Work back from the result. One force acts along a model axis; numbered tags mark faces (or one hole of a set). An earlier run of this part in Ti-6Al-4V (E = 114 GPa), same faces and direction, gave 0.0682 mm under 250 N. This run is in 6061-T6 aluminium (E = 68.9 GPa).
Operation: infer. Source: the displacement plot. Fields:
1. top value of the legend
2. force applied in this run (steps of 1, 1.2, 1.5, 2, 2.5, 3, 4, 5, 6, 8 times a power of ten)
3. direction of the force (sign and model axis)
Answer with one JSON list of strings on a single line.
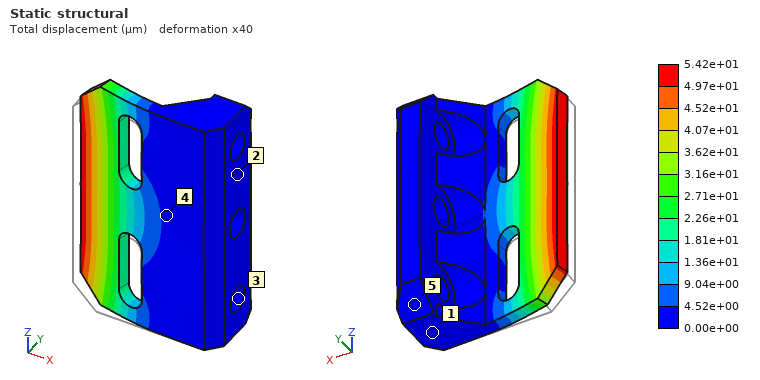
["5.42e+01 µm", "120 N", "+Y"]
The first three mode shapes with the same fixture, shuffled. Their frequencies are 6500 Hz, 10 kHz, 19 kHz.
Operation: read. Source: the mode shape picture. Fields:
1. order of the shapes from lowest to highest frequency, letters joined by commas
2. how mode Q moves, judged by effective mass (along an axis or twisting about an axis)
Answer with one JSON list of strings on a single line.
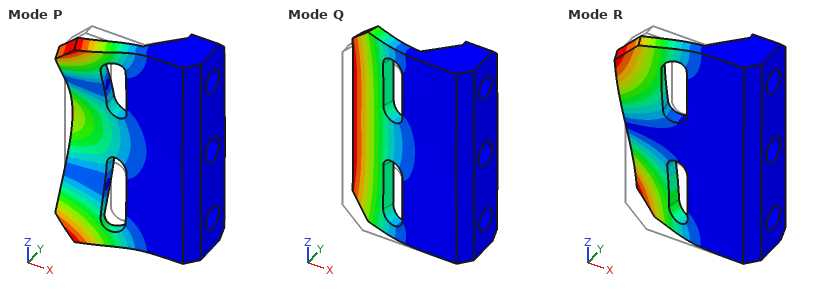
["Q, R, P", "along Y"]
